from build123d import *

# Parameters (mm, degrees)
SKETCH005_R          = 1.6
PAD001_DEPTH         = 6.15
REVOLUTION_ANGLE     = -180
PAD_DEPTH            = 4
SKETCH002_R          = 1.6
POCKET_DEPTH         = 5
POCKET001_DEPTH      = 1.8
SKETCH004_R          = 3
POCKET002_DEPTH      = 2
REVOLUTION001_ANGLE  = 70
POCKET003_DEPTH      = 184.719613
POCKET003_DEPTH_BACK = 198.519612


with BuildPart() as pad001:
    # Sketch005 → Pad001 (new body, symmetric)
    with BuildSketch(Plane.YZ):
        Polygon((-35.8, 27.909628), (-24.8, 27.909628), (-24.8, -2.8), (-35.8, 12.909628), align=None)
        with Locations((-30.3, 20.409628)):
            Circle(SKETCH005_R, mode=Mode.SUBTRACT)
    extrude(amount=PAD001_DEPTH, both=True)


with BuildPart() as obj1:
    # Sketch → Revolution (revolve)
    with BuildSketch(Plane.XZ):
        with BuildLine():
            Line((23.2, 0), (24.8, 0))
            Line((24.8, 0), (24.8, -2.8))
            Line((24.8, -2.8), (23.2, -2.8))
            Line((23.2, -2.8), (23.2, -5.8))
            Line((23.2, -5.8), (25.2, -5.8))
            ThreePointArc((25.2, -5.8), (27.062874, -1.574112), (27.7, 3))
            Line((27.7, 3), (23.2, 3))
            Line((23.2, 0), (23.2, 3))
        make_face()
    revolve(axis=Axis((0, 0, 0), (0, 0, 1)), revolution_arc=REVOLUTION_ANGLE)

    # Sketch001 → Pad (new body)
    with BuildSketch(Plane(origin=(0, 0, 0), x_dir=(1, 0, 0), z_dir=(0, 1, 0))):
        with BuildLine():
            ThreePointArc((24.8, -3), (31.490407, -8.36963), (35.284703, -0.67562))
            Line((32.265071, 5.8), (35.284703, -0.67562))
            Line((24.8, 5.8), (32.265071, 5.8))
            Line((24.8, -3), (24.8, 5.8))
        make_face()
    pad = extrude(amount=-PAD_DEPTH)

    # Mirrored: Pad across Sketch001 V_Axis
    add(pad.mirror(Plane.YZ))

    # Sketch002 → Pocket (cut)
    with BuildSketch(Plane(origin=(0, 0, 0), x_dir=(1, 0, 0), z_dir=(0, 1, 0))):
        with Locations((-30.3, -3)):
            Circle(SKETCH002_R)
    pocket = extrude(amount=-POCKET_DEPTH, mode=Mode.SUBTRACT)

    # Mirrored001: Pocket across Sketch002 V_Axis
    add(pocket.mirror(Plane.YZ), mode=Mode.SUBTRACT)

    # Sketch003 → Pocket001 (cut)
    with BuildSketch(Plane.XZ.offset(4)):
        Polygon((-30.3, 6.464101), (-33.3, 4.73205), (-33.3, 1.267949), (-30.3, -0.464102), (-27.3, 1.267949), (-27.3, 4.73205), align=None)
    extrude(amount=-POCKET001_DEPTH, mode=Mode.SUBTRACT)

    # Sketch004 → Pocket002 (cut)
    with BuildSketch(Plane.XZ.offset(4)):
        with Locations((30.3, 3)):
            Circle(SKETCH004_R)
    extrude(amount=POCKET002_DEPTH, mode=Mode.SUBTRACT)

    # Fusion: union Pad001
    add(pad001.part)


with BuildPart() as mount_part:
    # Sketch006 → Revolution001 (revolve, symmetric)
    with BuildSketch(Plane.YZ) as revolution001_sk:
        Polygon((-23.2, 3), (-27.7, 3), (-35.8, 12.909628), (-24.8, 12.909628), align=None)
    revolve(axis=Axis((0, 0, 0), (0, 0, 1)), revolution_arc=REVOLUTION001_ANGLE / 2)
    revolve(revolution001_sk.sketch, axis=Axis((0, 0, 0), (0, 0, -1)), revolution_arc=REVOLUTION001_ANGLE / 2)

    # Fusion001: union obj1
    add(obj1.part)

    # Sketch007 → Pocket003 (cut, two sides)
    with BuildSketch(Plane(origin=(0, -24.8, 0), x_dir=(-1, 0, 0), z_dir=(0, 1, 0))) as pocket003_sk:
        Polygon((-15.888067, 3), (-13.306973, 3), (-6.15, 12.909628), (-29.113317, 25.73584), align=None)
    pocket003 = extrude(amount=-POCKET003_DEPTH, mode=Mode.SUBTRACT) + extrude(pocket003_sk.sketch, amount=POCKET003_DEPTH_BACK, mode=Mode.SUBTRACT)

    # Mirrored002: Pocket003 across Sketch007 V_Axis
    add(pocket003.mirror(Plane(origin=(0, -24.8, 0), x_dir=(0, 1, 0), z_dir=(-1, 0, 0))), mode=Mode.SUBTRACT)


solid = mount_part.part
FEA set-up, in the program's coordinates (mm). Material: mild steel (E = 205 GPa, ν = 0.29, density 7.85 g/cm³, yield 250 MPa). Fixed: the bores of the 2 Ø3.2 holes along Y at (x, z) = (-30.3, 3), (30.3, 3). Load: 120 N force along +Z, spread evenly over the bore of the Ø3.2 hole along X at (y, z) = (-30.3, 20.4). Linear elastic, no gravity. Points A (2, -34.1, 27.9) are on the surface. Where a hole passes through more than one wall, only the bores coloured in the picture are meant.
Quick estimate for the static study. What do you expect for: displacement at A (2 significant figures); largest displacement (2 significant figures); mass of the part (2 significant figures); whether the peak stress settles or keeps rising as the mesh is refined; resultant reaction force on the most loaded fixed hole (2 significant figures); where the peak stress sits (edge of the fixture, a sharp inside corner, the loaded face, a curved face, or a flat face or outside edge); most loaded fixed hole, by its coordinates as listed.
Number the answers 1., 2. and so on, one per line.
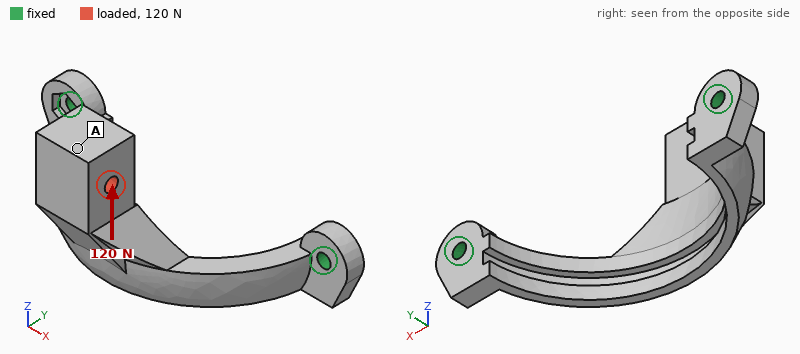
1. 84 µm
2. 87 µm
3. 51 g
4. keeps rising
5. 66 N
6. edge of the fixture
7. (30.3, 3)
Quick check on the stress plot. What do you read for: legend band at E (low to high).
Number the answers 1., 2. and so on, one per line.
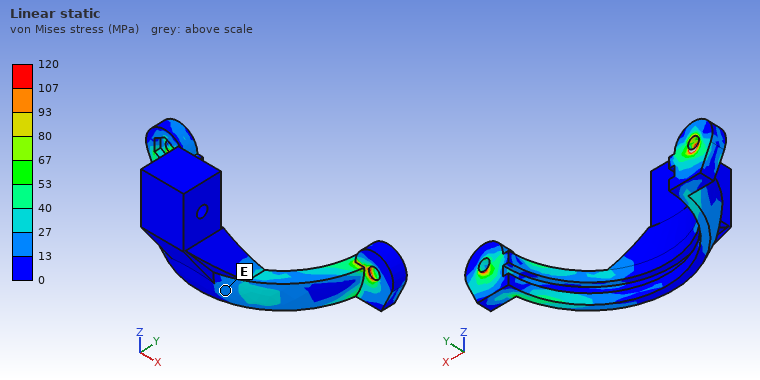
1. 13 to 27 MPa
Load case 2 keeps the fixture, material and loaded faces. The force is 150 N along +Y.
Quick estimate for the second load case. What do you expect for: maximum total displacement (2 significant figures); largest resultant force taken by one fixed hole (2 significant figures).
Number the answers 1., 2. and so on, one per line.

1. 0.12 mm
2. 92 N
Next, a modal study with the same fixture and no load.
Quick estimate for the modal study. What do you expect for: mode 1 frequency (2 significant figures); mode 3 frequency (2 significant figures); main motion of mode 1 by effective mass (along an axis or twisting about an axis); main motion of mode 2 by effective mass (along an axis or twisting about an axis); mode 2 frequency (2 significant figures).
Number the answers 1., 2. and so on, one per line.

1. 1200 Hz
2. 3800 Hz
3. along Z
4. along X
5. 3100 Hz
